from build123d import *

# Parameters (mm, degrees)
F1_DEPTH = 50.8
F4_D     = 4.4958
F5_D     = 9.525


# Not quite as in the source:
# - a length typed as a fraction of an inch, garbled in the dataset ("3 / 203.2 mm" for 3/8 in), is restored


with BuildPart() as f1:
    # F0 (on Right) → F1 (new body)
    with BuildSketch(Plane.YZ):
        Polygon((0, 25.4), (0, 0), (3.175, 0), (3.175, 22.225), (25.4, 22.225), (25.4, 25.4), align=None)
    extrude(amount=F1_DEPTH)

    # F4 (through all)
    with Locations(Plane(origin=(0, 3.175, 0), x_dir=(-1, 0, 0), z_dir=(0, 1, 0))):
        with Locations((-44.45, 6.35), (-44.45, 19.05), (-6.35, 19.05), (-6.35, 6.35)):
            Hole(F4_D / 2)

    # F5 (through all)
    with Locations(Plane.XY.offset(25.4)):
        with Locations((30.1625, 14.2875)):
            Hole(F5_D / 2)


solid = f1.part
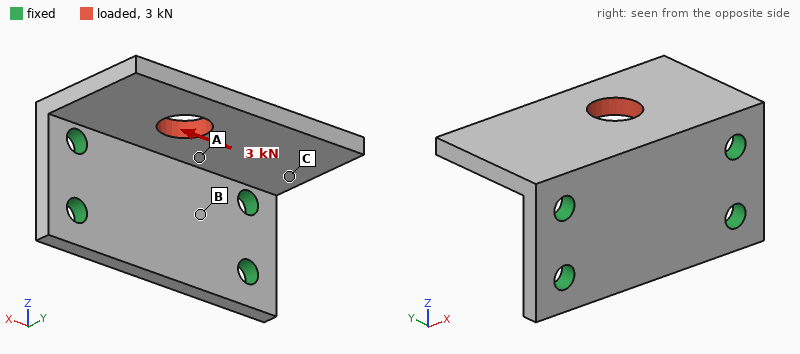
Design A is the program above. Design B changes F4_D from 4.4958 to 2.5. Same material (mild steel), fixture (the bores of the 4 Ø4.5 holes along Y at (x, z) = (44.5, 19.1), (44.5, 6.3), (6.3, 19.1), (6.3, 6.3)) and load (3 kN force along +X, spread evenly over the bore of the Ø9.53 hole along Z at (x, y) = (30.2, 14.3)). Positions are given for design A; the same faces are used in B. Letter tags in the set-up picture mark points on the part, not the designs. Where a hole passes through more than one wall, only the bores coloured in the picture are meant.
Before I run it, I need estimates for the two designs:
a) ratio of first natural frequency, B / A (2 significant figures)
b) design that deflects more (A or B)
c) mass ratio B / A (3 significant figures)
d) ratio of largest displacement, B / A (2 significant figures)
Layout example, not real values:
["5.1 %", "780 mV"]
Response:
["0.93", "B", "1.02", "1.5"]
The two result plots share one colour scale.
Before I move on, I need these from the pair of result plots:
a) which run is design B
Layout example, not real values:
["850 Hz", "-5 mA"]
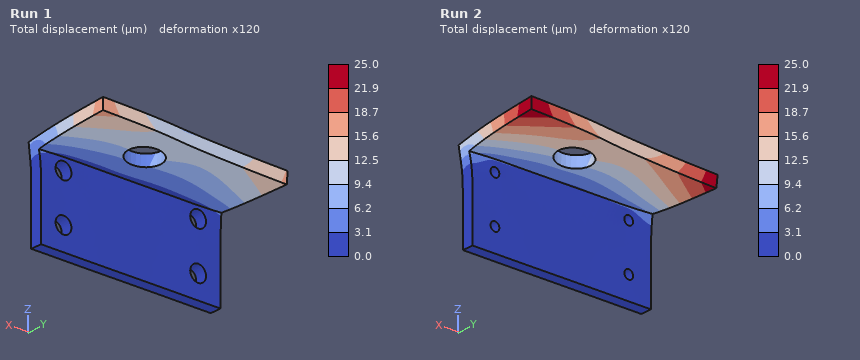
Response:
["Run 2"]
